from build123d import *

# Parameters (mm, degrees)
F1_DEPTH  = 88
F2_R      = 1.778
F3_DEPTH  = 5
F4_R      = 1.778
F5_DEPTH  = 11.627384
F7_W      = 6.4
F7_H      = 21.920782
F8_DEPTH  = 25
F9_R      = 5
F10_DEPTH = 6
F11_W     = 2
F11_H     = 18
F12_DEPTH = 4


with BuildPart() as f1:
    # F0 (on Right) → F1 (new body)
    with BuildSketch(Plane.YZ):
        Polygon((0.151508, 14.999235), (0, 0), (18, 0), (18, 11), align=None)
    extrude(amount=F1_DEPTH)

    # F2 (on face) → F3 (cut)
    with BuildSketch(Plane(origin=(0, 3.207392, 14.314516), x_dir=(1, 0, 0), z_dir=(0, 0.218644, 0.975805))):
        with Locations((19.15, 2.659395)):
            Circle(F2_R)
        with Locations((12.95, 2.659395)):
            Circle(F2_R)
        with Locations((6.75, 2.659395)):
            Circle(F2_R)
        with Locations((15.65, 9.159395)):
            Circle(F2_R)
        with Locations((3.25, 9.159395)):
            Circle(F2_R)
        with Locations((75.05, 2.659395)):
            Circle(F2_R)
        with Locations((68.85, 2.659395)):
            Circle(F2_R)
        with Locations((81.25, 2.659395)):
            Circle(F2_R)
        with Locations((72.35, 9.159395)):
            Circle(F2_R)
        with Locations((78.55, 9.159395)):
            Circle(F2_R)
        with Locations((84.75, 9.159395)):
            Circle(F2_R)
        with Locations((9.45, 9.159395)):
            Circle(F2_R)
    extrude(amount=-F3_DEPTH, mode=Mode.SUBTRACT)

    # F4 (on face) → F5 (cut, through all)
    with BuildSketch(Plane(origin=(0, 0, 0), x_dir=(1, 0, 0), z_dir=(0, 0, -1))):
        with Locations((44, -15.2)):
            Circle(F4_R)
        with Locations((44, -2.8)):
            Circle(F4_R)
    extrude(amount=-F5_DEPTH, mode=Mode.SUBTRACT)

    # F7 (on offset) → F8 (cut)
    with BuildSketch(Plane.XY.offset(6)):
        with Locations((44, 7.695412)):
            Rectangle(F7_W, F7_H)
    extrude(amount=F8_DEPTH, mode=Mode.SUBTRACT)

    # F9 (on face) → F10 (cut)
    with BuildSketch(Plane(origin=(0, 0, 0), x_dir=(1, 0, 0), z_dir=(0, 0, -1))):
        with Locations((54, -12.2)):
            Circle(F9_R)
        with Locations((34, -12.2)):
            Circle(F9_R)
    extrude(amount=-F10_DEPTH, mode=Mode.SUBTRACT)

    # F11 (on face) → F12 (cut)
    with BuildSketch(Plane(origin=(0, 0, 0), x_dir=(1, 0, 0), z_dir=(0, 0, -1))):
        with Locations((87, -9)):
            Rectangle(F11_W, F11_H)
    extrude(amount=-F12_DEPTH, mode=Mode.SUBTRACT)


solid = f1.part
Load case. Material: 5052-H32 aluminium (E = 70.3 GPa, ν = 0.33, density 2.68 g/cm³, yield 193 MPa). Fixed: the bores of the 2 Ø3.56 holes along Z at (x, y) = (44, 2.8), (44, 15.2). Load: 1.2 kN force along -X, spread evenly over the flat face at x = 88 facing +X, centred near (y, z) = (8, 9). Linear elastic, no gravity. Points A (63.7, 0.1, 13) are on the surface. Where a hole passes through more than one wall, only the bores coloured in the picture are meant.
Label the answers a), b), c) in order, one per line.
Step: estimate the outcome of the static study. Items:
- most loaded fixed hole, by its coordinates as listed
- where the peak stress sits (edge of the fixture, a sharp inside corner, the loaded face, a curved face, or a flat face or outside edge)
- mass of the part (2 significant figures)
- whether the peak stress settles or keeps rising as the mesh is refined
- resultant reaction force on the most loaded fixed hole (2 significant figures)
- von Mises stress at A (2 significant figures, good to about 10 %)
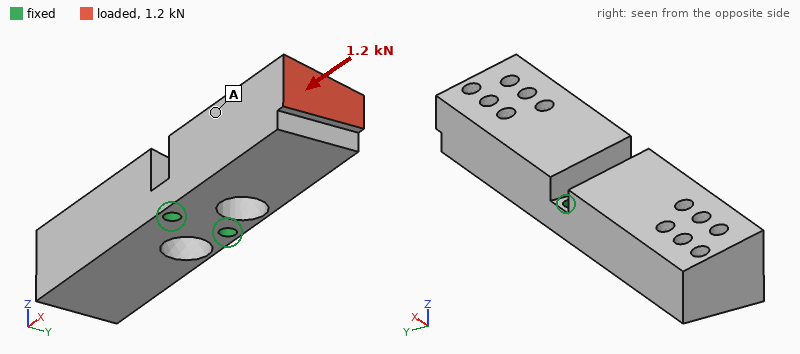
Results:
a) (44, 2.8)
b) edge of the fixture
c) 48 g
d) keeps rising
e) 670 N
f) 11 MPa
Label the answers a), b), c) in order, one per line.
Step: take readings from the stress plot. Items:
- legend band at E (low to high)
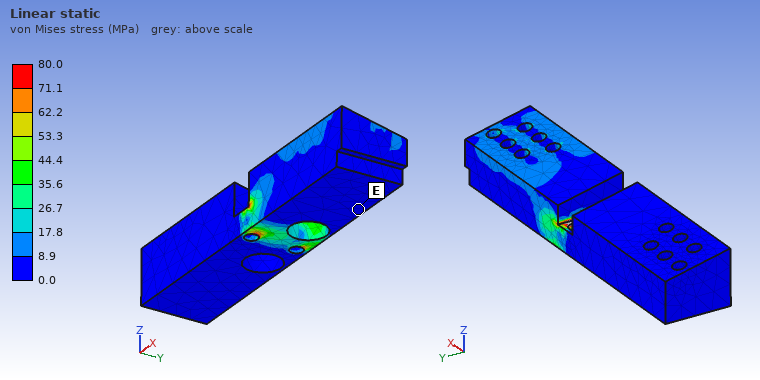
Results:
a) 0.0 to 8.9 MPa
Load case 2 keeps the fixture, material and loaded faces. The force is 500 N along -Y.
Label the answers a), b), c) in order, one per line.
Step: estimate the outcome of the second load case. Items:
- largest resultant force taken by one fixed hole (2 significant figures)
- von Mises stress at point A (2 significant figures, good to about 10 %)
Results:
a) 1.6 kN
b) 15 MPa
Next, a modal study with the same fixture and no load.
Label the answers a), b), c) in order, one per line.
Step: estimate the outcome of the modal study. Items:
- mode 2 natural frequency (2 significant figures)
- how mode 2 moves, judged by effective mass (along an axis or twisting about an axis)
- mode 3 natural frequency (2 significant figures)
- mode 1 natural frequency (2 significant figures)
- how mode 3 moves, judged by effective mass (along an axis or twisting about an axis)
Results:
a) 2400 Hz
b) along Z
c) 4800 Hz
d) 2200 Hz
e) along Y
